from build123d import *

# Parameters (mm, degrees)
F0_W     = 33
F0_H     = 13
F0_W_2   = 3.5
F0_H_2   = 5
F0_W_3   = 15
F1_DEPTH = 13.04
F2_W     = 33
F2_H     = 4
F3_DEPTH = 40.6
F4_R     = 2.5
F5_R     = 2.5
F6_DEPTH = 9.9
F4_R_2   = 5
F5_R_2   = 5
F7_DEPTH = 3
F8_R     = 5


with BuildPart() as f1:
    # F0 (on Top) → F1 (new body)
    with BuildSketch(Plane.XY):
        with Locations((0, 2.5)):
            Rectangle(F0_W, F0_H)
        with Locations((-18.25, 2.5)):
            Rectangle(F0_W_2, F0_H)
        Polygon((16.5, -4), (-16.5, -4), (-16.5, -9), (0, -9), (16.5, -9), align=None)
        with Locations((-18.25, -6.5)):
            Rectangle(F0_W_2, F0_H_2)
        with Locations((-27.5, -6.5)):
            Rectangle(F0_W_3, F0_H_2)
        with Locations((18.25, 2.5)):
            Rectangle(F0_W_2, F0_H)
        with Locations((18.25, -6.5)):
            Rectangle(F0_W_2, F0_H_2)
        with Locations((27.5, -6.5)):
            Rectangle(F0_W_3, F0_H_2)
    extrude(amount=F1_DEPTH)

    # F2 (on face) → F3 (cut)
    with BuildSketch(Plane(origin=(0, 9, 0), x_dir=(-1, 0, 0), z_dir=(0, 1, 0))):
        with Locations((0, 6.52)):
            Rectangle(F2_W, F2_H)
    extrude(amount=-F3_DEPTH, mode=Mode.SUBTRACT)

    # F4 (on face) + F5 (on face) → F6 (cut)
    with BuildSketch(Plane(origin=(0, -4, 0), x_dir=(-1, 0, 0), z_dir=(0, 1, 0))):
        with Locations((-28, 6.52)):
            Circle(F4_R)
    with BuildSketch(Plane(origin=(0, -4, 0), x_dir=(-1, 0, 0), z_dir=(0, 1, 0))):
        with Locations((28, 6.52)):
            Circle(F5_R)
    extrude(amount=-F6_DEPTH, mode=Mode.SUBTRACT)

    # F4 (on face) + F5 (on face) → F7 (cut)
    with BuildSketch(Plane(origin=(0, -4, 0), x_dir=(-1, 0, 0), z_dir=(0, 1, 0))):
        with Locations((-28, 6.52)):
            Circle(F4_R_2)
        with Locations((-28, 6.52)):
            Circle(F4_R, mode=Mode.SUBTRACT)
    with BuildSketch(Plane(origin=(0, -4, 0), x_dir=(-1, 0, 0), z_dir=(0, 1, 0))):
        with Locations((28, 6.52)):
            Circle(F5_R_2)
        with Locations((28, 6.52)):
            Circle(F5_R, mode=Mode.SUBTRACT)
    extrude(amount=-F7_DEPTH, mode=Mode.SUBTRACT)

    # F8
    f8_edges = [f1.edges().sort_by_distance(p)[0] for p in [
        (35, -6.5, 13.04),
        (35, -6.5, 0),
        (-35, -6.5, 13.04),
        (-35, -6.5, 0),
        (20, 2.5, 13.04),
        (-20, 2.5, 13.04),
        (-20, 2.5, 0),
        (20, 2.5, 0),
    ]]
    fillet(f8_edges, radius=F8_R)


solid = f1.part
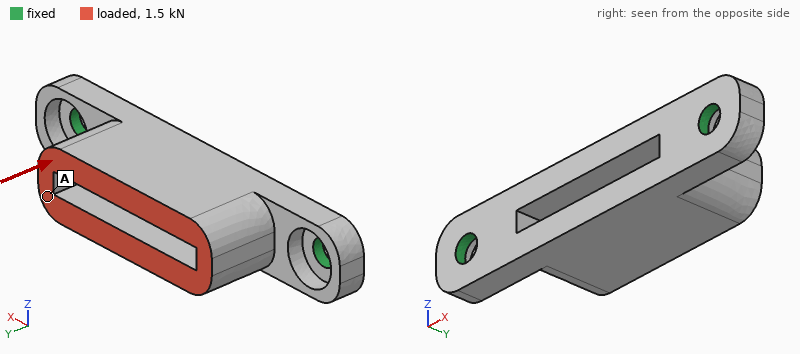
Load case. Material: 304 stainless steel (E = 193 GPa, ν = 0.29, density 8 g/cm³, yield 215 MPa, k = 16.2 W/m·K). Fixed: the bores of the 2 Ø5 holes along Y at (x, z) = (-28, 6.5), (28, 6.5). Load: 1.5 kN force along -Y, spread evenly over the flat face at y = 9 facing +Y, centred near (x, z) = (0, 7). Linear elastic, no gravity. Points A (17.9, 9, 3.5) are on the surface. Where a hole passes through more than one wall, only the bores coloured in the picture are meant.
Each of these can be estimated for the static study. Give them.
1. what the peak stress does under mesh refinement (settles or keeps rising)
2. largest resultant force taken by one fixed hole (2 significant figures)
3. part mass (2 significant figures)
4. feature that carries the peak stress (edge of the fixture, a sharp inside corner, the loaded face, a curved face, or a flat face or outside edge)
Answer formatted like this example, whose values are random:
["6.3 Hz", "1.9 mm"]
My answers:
["keeps rising", "1.1 kN", "64 g", "edge of the fixture"]
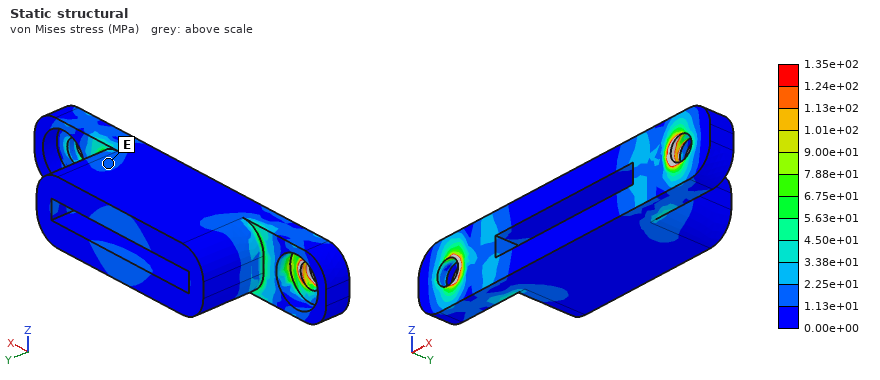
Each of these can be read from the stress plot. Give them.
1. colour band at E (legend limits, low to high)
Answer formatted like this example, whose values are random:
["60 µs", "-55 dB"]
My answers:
["1.13e+01 to 2.25e+01 MPa"]
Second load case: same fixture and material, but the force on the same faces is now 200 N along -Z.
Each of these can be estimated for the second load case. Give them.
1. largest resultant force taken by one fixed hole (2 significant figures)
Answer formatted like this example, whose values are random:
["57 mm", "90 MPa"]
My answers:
["100 N"]
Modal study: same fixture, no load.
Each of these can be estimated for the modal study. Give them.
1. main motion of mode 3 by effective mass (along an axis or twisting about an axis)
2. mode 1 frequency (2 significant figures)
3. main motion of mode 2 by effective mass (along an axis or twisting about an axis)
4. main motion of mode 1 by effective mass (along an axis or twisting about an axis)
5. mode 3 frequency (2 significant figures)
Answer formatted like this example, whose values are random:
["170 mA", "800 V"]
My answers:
["twisting about Y", "3700 Hz", "along Y", "along Z", "12 kHz"]
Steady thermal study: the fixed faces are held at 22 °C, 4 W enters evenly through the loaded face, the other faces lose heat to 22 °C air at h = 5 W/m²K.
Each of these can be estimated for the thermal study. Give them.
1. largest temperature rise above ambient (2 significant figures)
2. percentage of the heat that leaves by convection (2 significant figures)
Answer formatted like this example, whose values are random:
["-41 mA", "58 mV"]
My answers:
["38 K", "14 %"]
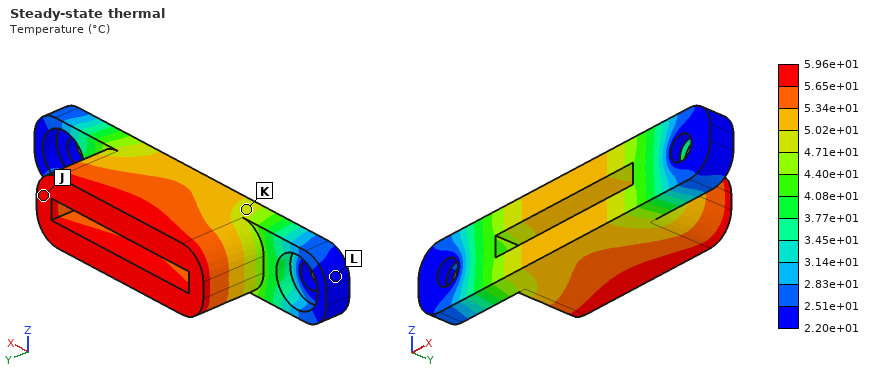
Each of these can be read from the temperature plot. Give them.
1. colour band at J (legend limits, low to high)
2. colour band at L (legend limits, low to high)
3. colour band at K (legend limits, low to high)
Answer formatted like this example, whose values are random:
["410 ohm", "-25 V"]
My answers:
["5.65e+01 to 5.96e+01 °C", "2.20e+01 to 2.51e+01 °C", "4.71e+01 to 5.02e+01 °C"]
